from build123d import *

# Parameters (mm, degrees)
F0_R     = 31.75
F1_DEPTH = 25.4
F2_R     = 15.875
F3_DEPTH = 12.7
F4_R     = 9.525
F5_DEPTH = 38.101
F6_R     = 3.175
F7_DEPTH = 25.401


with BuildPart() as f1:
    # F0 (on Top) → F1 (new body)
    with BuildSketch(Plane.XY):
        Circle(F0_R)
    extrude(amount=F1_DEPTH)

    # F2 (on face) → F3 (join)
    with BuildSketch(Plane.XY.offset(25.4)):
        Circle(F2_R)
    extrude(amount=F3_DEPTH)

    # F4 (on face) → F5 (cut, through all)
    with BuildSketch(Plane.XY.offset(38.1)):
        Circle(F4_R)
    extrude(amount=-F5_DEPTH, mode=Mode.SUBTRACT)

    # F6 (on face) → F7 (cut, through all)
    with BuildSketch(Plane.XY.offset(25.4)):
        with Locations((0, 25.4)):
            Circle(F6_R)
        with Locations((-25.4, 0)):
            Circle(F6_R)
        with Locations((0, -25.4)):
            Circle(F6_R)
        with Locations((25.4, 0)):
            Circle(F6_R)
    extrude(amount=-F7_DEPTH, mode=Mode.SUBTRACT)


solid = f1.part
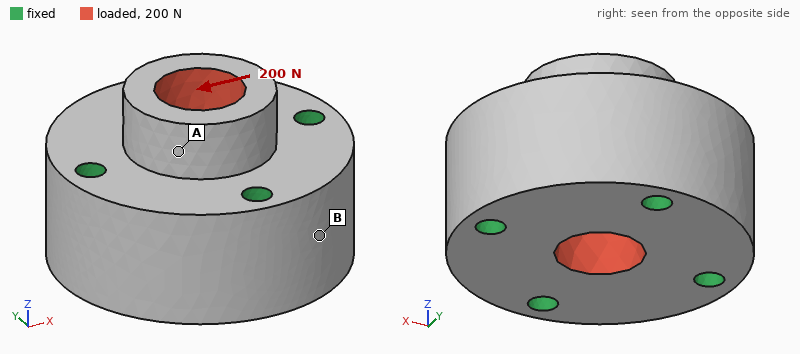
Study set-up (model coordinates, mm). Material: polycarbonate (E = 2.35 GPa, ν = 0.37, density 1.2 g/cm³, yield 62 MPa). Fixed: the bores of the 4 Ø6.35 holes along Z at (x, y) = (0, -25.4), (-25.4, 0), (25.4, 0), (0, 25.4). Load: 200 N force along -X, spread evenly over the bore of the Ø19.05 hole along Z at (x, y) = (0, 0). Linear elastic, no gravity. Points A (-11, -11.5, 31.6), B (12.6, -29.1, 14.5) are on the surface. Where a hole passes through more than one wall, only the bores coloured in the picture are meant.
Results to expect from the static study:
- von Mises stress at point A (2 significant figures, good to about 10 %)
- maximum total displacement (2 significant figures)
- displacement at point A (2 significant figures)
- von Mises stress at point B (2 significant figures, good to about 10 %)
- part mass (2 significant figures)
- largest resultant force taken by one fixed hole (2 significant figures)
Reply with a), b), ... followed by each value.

a) 0.12 MPa
b) 4.6 µm
c) 2.8 µm
d) 0.043 MPa
e) 92 g
f) 67 N
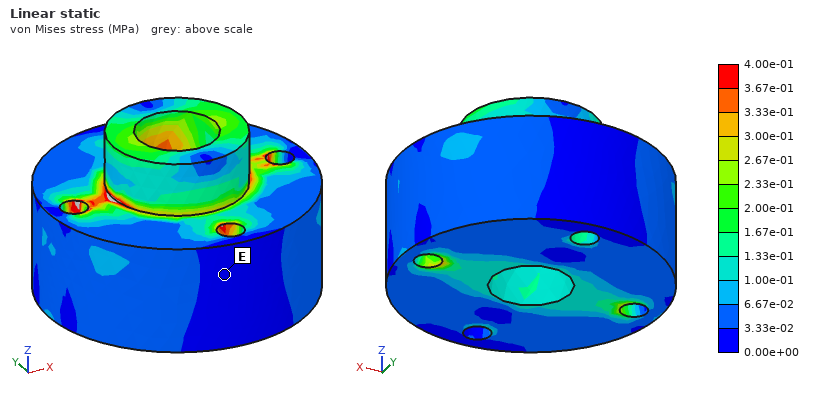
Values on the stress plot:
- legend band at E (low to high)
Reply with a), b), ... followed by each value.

a) 0.00e+00 to 3.33e-02 MPa
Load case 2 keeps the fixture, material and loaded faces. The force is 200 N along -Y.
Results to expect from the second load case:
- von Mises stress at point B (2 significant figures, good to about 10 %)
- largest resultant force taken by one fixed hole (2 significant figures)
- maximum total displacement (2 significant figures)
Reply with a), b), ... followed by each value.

a) 0.060 MPa
b) 67 N
c) 4.6 µm
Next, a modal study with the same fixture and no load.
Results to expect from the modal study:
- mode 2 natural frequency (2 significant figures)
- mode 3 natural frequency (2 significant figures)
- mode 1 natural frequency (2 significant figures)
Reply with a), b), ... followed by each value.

a) 8100 Hz
b) 8600 Hz
c) 8100 Hz
